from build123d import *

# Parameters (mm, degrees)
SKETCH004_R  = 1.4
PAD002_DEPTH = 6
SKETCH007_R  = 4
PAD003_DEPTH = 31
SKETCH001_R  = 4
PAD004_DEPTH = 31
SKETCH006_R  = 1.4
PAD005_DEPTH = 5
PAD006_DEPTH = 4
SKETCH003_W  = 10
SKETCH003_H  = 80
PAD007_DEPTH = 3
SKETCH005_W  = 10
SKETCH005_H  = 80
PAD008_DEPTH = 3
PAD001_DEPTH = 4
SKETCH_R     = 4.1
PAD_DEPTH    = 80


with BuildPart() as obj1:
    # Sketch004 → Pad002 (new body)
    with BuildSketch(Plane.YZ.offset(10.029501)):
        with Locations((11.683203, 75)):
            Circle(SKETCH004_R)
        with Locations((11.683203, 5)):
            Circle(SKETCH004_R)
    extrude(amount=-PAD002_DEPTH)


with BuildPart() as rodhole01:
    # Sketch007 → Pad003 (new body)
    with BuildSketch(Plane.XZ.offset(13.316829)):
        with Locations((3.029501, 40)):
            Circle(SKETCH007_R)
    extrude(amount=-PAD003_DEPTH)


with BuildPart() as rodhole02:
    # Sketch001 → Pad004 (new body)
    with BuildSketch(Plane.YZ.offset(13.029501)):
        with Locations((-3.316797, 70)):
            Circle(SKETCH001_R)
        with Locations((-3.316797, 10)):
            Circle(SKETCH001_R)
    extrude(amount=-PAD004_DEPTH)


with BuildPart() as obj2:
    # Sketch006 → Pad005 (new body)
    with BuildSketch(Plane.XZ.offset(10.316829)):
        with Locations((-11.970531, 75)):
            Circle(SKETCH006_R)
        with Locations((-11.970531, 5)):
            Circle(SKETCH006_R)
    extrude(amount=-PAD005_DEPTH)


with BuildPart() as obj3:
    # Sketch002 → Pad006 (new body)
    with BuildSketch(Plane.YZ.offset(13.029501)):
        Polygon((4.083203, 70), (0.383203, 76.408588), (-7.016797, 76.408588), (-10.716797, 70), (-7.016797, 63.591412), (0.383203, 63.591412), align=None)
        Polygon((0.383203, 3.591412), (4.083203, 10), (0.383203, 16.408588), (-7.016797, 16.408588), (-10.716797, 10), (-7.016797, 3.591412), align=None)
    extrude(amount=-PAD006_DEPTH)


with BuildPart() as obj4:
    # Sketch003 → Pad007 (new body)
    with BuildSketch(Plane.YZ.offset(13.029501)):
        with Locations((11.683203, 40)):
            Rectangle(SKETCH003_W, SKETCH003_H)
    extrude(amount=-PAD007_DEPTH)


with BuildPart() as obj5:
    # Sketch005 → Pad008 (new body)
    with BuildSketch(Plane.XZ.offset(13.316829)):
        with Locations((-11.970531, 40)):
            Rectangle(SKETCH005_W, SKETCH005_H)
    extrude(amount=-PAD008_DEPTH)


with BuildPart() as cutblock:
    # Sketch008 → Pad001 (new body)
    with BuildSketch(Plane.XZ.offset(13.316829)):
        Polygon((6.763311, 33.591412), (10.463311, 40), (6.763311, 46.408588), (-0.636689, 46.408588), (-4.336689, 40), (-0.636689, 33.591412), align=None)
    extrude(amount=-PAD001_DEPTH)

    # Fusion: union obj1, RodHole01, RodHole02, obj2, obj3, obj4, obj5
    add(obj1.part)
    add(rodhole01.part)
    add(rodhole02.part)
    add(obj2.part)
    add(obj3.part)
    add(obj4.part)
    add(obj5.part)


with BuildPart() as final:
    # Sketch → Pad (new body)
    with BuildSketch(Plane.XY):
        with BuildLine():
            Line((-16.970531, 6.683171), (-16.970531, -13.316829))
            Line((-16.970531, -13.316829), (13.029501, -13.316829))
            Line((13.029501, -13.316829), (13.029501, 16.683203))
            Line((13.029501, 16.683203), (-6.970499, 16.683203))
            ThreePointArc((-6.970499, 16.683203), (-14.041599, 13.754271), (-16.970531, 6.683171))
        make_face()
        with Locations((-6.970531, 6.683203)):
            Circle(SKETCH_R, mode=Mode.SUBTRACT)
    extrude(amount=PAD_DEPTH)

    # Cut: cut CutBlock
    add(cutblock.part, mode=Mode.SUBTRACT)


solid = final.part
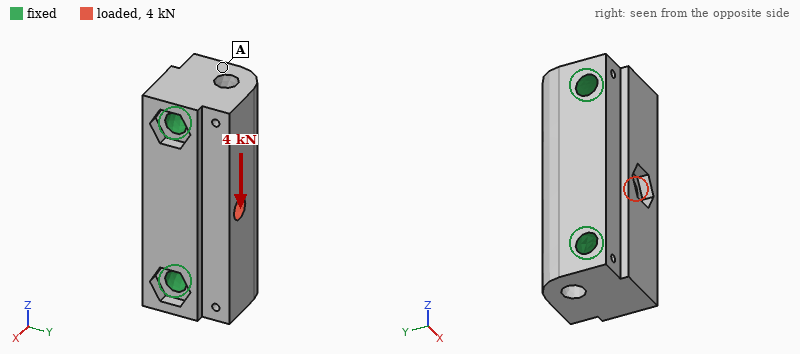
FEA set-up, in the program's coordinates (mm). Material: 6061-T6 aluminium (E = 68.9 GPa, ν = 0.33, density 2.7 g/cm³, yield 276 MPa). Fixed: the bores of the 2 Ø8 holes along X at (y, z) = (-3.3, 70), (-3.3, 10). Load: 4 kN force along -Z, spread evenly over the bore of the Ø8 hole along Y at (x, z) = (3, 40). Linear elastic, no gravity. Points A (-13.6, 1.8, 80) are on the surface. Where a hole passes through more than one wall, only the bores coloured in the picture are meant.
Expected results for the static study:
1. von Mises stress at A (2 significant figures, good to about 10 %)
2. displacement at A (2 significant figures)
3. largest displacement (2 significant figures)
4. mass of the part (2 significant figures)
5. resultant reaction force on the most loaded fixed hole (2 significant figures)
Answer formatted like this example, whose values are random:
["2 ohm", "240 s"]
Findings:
["1.8 MPa", "0.39 µm", "2.5 µm", "150 g", "2.1 kN"]
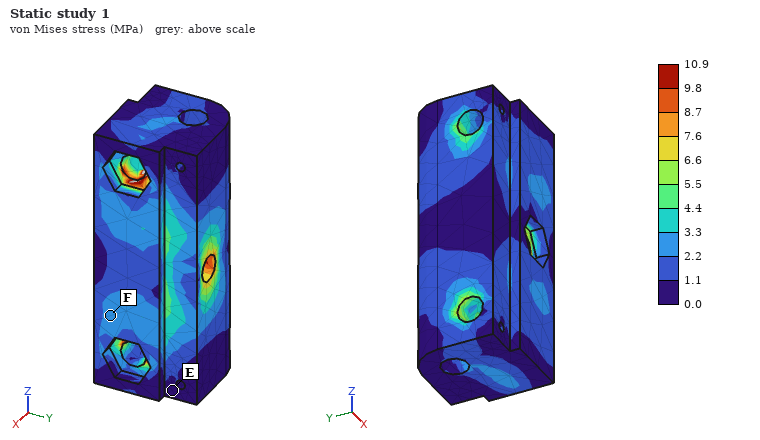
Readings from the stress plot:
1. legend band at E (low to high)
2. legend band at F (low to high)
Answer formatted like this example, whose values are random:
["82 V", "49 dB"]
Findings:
["0.0 to 1.1 MPa", "2.2 to 3.3 MPa"]
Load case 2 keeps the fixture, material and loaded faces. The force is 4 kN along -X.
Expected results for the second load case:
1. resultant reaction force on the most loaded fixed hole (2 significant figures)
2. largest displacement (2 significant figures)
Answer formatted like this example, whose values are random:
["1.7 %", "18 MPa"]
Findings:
["2.0 kN", "9.1 µm"]
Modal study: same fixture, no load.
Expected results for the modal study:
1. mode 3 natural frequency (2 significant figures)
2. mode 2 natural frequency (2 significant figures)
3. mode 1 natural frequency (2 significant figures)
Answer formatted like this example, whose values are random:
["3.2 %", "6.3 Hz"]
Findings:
["23 kHz", "18 kHz", "17 kHz"]
